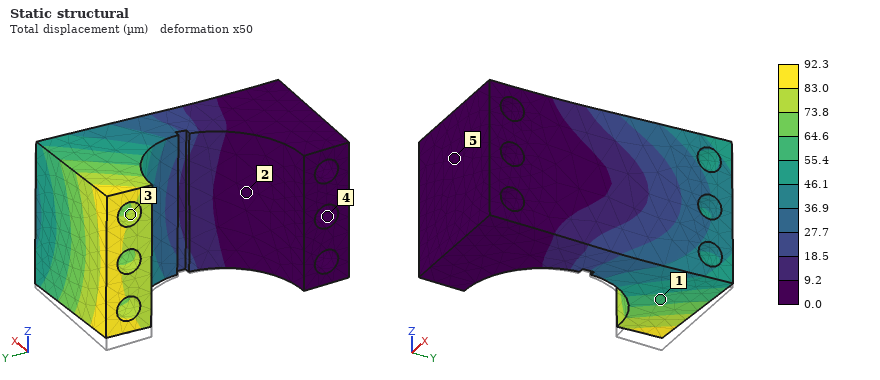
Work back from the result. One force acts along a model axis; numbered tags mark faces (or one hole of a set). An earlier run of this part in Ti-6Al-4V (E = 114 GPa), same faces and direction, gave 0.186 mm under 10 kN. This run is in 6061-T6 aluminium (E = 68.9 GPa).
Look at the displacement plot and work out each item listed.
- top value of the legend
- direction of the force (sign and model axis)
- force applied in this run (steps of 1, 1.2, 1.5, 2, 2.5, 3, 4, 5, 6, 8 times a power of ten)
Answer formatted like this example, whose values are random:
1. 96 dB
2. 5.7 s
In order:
1. 92.3 µm
2. +Z
3. 3 kN
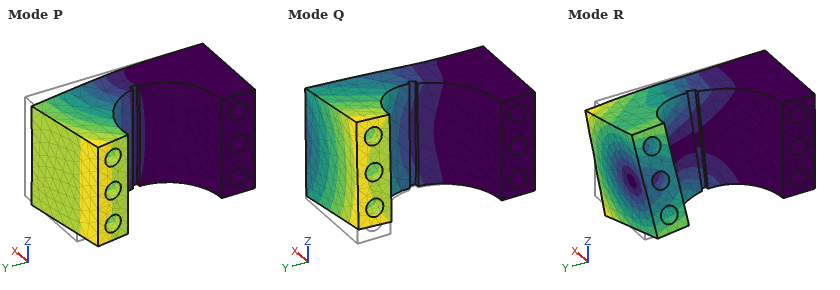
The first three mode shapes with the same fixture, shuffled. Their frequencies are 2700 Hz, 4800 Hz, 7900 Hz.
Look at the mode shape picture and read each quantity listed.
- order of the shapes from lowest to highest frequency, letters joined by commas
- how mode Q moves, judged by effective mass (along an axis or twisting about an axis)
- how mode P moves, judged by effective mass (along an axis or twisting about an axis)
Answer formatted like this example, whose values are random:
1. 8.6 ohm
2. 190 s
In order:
1. P, Q, R
2. along Z
3. along X
